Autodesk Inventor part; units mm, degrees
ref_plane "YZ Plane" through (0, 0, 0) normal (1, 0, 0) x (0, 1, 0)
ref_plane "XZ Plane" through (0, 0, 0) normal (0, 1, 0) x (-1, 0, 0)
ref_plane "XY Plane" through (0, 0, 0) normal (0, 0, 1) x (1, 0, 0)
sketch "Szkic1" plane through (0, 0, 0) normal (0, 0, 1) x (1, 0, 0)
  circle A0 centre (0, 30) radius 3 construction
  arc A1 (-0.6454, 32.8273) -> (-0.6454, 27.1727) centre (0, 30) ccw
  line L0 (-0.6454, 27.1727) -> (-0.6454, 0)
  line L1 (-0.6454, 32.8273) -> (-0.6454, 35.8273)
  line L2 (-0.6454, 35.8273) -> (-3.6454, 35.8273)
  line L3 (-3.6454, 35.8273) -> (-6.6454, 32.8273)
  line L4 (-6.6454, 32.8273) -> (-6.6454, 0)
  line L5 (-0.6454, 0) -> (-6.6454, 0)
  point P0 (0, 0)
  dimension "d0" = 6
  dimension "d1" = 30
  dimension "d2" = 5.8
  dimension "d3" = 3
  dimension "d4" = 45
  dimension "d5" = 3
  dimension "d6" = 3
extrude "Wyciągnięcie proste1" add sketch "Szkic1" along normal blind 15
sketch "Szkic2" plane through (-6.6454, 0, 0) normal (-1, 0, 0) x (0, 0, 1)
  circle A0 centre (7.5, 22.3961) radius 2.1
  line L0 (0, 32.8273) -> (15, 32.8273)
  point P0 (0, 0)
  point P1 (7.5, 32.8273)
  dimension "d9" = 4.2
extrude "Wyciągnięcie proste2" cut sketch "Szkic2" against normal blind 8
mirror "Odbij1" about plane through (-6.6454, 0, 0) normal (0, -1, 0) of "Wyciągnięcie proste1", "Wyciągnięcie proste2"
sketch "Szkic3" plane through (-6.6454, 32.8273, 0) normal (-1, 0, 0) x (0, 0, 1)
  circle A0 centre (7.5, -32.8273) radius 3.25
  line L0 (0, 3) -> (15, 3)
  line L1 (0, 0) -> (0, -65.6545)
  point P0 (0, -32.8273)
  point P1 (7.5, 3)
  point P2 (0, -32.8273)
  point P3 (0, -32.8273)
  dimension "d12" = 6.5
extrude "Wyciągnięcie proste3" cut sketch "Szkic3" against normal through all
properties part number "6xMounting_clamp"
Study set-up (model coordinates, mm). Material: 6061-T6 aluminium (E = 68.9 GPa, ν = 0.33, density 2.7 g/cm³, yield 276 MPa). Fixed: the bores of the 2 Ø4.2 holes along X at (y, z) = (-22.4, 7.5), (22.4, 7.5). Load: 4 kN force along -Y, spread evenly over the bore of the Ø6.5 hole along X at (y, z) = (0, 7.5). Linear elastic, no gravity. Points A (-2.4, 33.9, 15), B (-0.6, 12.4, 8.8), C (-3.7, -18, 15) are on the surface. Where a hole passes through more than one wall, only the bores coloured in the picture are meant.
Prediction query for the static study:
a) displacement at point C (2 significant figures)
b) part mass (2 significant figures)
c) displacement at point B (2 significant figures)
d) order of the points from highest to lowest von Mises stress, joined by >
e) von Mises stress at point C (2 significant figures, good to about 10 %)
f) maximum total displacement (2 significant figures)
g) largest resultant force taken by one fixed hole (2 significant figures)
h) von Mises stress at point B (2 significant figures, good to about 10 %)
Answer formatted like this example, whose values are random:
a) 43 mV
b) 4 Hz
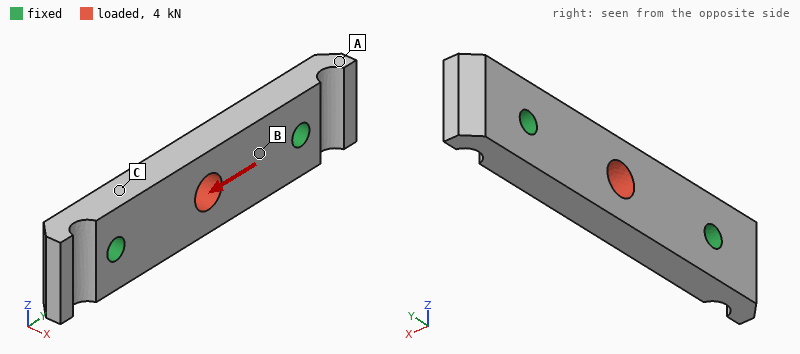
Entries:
a) 2.7 µm
b) 15 g
c) 3.7 µm
d) B > C > A
e) 12 MPa
f) 8.3 µm
g) 2.0 kN
h) 27 MPa
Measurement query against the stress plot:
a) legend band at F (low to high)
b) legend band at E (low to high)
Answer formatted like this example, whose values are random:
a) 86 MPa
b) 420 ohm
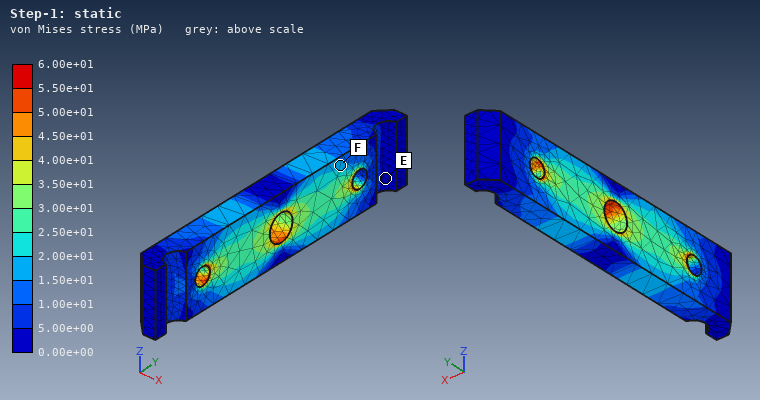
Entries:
a) 1.50e+01 to 2.00e+01 MPa
b) 0.00e+00 to 5.00e+00 MPa
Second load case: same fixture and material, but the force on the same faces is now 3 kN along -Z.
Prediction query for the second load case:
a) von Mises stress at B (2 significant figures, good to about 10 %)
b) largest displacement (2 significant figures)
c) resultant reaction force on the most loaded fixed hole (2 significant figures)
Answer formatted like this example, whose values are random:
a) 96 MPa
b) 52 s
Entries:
a) 42 MPa
b) 38 µm
c) 1.5 kN
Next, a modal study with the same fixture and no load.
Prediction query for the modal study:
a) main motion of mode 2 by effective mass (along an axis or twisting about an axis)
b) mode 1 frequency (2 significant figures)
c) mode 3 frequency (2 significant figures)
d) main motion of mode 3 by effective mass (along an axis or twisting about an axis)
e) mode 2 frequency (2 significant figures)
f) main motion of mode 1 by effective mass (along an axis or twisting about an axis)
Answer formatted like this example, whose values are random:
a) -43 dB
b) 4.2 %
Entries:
a) along Z
b) 14 kHz
c) 23 kHz
d) twisting about Y
e) 20 kHz
f) along X
